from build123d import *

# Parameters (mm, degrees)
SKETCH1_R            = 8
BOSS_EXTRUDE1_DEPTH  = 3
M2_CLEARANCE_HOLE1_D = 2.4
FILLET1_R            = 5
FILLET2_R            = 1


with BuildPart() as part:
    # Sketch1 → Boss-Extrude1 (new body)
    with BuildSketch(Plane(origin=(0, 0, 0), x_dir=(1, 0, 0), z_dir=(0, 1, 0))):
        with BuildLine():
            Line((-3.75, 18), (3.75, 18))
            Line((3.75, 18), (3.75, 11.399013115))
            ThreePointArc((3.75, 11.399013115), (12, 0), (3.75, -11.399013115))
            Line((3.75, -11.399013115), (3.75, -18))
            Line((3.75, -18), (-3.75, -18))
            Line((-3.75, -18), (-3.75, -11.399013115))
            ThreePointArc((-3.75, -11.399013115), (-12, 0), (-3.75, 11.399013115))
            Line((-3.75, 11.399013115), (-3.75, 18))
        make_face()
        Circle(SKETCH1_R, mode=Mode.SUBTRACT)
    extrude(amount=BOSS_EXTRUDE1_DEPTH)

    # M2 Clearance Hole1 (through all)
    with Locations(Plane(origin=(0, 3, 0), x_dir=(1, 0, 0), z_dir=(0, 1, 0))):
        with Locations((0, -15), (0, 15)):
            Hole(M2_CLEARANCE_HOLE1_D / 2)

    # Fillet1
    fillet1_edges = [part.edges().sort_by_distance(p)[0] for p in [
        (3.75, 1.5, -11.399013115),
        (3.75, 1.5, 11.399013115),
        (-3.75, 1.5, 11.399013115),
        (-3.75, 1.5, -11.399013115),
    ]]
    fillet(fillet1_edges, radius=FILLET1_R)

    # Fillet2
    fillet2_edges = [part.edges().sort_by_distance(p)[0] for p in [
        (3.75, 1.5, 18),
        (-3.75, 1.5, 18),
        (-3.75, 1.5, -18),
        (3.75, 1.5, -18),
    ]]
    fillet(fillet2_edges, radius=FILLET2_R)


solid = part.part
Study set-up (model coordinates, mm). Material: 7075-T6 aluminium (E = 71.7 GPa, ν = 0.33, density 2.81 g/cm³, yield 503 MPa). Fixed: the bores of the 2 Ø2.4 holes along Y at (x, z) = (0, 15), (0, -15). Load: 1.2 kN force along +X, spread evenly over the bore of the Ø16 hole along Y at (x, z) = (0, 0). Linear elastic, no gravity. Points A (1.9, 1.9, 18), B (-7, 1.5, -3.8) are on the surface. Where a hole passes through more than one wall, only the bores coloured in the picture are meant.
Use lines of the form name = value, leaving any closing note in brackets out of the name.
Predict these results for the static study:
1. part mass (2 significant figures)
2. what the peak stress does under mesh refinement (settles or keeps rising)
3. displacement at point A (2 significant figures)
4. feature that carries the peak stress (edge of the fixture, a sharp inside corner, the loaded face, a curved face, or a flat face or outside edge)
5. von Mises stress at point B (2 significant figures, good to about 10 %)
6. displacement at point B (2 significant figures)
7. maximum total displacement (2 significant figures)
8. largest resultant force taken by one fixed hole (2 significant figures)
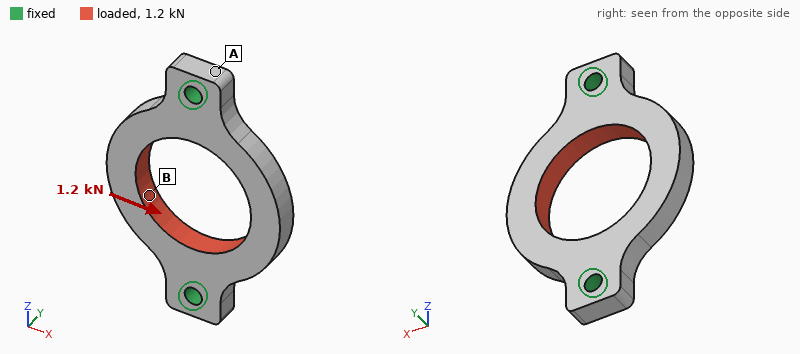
part mass = 2.9 g
what the peak stress does under mesh refinement = keeps rising
displacement at point A = 1.5 µm
feature that carries the peak stress = edge of the fixture
von Mises stress at point B = 29 MPa
displacement at point B = 10.0 µm
maximum total displacement = 10 µm
largest resultant force taken by one fixed hole = 600 N
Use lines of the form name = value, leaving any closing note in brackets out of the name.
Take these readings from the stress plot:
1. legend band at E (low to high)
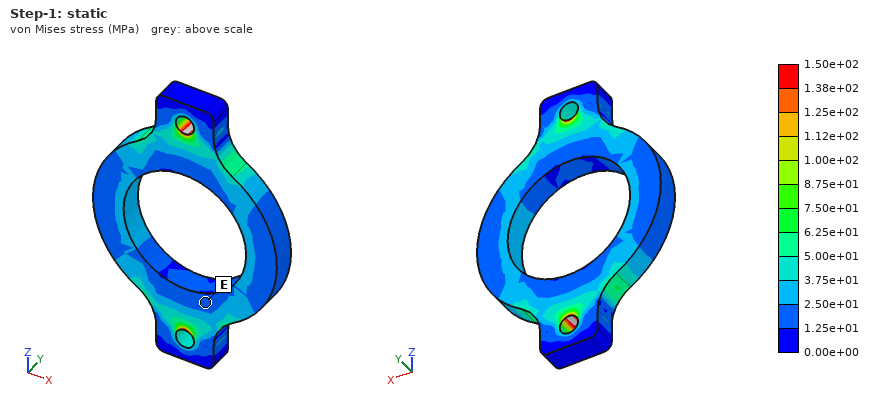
legend band at E = 1.25e+01 to 2.50e+01 MPa
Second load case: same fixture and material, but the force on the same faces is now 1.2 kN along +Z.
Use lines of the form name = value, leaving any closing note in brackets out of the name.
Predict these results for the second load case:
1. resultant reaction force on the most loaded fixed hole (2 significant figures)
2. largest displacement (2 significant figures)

resultant reaction force on the most loaded fixed hole = 600 N
largest displacement = 8.5 µm
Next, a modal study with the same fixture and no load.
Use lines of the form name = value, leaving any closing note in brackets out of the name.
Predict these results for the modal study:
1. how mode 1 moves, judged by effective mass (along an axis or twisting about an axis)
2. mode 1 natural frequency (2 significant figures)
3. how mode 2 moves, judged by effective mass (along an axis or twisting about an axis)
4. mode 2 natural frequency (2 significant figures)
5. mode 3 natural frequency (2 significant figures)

how mode 1 moves, judged by effective mass = twisting about Z
mode 1 natural frequency = 10 kHz
how mode 2 moves, judged by effective mass = along Y
mode 2 natural frequency = 12 kHz
mode 3 natural frequency = 28 kHz
